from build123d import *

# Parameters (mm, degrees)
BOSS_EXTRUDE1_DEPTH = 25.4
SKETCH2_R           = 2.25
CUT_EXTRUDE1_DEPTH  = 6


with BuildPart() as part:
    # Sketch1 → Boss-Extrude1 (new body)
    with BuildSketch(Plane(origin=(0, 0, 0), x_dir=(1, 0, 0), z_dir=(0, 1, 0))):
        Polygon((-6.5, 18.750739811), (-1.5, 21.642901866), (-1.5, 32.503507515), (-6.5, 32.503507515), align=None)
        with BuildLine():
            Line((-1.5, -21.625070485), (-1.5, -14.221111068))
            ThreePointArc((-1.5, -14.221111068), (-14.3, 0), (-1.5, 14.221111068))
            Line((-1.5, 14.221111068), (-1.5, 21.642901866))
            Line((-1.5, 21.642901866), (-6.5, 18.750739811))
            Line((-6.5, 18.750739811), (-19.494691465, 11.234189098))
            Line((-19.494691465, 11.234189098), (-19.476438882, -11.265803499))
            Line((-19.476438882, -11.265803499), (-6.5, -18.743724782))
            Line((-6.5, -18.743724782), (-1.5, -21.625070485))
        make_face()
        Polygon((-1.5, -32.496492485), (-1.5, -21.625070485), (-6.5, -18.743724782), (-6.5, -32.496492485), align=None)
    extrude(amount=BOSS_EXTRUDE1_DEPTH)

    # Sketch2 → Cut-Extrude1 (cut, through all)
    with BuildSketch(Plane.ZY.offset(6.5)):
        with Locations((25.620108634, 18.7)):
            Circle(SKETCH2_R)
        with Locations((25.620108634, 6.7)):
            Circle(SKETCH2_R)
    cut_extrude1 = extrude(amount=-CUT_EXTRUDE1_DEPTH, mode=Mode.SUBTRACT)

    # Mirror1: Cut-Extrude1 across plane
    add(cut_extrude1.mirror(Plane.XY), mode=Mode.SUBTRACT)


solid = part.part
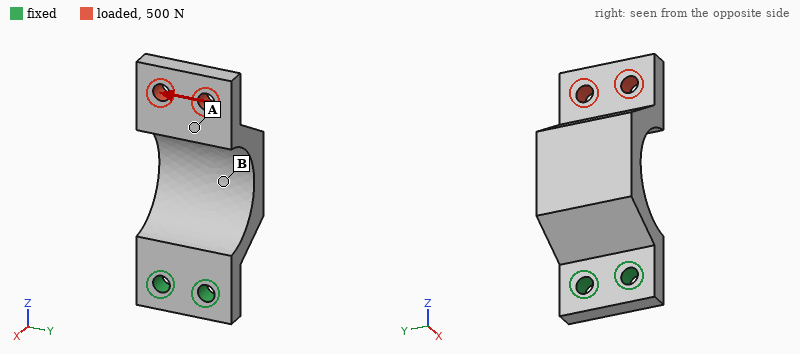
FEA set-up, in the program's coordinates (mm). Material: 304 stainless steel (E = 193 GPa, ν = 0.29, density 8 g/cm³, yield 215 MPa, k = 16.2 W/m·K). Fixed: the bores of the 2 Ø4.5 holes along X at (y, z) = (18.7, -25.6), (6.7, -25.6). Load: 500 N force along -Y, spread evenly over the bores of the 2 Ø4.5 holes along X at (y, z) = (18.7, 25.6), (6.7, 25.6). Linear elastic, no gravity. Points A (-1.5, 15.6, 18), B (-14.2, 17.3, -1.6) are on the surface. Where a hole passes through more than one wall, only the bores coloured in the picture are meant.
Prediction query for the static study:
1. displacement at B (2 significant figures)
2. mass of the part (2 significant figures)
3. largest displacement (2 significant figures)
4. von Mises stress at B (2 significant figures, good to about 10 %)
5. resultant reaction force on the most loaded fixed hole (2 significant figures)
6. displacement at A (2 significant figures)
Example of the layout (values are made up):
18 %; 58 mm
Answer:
0.020 mm; 86 g; 0.12 mm; 62 MPa; 1.7 kN; 0.083 mm
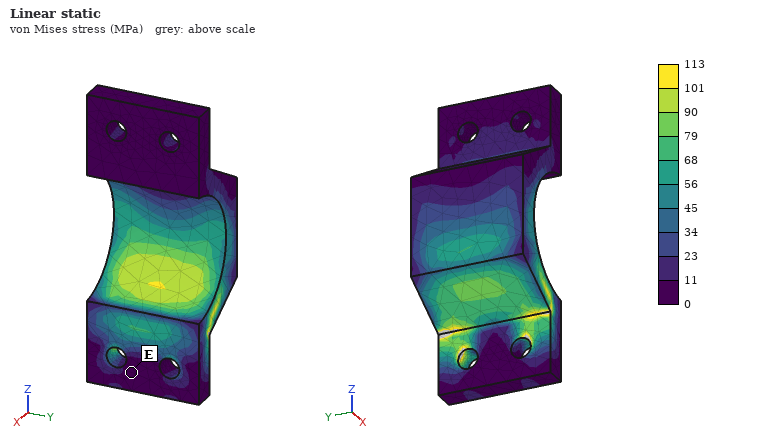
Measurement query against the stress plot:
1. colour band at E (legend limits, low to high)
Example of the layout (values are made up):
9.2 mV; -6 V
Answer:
0 to 11 MPa
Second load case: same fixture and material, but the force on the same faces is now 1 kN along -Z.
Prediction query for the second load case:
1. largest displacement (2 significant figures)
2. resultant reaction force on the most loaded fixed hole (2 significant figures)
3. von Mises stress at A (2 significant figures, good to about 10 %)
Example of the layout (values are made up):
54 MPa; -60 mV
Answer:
0.17 mm; 500 N; 11 MPa
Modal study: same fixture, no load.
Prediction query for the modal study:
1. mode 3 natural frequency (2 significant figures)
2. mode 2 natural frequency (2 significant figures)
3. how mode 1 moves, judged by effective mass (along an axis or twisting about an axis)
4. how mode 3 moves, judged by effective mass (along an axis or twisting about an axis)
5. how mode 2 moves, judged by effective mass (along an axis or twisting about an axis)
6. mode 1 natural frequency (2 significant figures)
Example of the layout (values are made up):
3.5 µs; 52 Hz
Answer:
4300 Hz; 2400 Hz; along X; along Z; along Y; 1100 Hz
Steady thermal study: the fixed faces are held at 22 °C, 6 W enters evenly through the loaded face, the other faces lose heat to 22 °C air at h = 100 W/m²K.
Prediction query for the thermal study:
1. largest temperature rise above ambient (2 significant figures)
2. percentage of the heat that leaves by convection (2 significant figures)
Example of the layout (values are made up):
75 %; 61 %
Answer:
40 K; 94 %
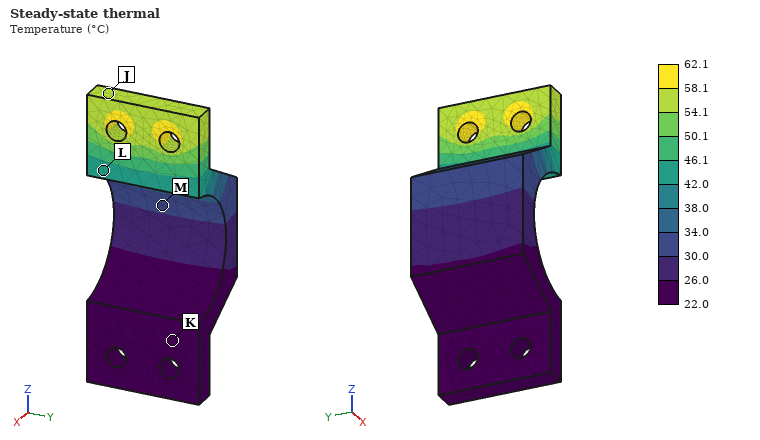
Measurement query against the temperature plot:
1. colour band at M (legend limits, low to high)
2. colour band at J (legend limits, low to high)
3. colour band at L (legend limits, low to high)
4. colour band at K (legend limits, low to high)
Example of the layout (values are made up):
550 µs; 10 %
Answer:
30.0 to 34.0 °C; 54.1 to 58.1 °C; 42.0 to 46.1 °C; 22.0 to 26.0 °C
